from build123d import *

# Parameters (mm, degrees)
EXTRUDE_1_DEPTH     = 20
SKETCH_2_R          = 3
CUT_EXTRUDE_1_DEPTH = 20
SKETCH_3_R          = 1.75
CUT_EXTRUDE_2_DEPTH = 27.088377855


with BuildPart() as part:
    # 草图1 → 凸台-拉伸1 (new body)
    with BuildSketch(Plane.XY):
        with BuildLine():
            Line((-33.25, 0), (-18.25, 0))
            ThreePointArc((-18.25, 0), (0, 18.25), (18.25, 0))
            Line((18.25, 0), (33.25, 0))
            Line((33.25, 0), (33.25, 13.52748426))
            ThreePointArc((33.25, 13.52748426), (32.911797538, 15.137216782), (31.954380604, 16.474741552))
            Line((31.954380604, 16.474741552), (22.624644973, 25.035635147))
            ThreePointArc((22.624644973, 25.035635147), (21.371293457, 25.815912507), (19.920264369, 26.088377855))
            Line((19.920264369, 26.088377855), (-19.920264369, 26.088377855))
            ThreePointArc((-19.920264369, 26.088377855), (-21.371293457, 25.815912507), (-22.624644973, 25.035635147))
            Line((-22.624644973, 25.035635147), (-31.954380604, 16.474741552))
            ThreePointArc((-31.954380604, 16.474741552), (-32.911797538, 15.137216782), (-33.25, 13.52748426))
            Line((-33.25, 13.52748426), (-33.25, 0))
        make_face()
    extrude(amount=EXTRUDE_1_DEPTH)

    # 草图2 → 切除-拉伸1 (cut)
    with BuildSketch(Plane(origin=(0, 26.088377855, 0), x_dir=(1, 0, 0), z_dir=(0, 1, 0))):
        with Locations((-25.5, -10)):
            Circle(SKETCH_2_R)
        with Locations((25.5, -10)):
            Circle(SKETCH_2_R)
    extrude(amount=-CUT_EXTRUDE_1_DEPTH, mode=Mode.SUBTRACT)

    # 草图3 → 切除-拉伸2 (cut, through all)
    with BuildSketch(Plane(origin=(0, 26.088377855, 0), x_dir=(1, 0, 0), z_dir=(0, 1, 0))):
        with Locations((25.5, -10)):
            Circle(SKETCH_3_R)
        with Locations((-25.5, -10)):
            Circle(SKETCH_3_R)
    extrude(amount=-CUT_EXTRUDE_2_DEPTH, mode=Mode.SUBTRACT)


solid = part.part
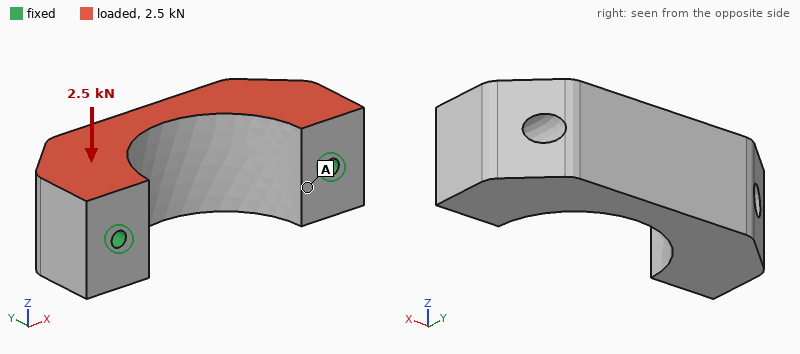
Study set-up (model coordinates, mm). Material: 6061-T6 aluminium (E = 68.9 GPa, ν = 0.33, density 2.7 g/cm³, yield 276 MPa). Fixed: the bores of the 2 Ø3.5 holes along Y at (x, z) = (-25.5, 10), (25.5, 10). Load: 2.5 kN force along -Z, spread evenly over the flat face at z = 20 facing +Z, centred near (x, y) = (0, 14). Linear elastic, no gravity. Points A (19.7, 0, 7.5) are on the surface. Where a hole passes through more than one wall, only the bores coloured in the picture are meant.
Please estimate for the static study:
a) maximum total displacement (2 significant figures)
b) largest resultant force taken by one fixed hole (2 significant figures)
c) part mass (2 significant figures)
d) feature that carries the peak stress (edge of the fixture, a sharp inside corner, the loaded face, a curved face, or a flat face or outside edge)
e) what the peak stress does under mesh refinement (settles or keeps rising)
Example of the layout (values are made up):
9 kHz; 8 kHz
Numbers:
53 µm; 1.3 kN; 56 g; edge of the fixture; keeps rising
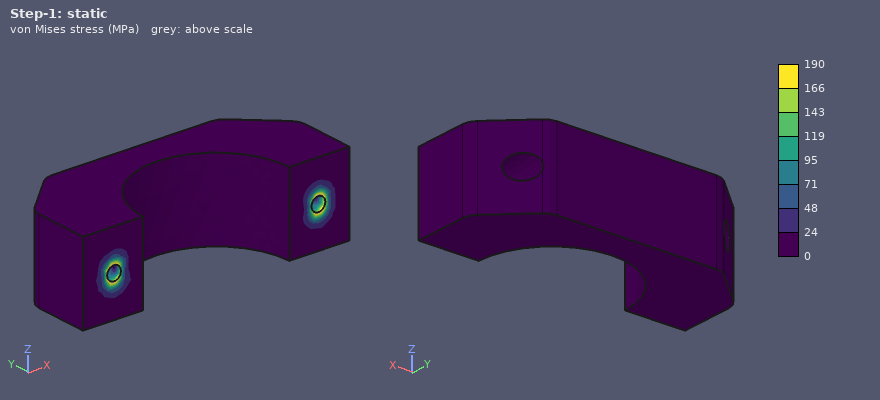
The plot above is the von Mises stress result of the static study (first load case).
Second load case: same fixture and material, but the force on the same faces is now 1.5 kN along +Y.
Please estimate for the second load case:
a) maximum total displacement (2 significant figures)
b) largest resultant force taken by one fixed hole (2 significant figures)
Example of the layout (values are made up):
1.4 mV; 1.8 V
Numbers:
27 µm; 780 N
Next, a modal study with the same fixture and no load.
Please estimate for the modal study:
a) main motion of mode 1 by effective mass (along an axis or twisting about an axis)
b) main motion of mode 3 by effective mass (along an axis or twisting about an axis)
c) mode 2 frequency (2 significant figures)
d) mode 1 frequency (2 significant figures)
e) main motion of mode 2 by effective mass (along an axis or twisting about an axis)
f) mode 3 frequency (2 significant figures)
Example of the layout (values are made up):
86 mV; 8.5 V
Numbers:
along Z; along X; 11 kHz; 5400 Hz; twisting about Y; 13 kHz
